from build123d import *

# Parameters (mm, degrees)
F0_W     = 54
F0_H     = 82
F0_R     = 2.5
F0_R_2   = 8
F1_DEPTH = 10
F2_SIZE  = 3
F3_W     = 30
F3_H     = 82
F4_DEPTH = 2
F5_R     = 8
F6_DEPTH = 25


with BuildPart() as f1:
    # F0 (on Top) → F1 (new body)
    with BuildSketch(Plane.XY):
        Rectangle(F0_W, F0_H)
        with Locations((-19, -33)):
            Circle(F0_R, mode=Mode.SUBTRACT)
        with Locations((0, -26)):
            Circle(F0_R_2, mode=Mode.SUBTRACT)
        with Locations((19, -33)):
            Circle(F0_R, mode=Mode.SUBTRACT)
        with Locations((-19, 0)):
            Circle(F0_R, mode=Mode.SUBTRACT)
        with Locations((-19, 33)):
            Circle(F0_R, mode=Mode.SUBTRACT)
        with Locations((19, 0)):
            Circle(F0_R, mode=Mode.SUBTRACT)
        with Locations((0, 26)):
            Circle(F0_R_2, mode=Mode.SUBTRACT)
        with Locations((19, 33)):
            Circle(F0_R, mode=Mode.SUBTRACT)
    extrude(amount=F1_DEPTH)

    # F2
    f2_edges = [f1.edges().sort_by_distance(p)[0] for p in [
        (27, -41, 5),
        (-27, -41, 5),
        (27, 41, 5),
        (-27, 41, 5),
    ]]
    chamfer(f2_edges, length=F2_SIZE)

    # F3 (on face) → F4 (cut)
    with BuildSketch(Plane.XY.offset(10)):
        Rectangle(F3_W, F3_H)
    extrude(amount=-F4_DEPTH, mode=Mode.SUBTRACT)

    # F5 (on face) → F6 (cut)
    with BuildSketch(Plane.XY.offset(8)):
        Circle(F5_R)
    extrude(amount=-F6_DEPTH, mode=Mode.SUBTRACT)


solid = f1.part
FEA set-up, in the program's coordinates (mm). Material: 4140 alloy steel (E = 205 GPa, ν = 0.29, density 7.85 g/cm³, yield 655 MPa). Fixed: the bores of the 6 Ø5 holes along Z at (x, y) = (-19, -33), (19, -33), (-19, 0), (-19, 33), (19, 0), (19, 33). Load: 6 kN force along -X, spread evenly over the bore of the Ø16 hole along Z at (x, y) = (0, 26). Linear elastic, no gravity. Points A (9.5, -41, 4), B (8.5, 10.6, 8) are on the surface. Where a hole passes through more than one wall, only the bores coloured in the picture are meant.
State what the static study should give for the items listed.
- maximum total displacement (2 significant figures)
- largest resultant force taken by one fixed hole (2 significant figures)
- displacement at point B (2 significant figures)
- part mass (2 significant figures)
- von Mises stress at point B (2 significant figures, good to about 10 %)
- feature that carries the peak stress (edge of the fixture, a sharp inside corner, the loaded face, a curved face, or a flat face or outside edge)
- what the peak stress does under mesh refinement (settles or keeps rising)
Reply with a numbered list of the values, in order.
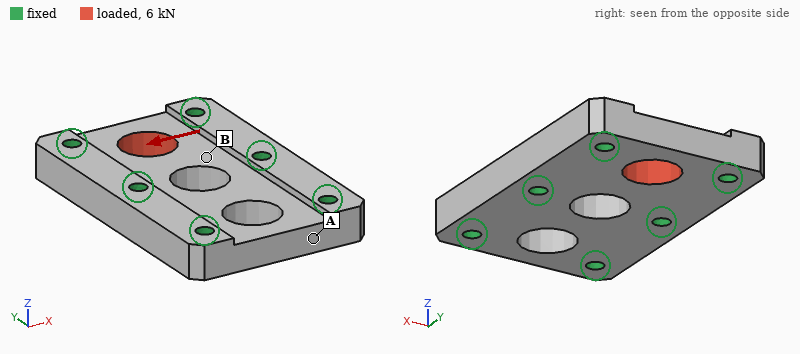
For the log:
1. 1.6 µm
2. 2.2 kN
3. 0.76 µm
4. 260 g
5. 8.3 MPa
6. edge of the fixture
7. keeps rising
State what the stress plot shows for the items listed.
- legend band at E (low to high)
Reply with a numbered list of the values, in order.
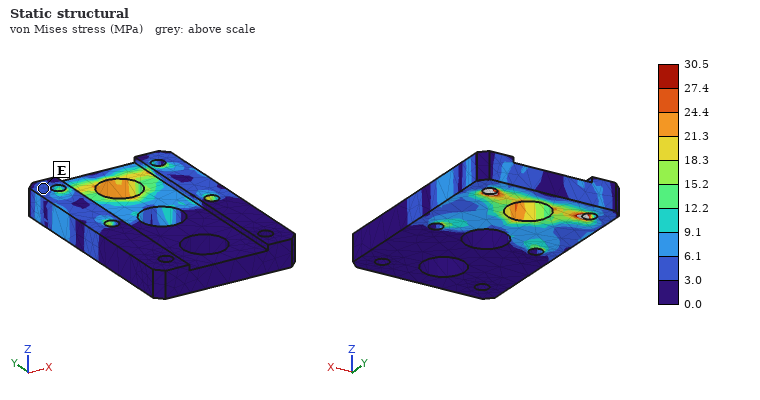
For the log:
1. 3.0 to 6.1 MPa
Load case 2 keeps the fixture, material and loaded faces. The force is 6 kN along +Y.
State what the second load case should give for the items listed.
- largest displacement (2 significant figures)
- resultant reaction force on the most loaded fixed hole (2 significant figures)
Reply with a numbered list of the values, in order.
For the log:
1. 3.9 µm
2. 1.8 kN
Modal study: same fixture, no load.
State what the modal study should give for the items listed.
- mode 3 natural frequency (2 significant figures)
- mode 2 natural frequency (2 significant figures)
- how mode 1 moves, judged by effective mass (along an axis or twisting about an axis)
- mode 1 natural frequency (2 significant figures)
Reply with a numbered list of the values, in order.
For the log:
1. 30 kHz
2. 24 kHz
3. along Z
4. 23 kHz
